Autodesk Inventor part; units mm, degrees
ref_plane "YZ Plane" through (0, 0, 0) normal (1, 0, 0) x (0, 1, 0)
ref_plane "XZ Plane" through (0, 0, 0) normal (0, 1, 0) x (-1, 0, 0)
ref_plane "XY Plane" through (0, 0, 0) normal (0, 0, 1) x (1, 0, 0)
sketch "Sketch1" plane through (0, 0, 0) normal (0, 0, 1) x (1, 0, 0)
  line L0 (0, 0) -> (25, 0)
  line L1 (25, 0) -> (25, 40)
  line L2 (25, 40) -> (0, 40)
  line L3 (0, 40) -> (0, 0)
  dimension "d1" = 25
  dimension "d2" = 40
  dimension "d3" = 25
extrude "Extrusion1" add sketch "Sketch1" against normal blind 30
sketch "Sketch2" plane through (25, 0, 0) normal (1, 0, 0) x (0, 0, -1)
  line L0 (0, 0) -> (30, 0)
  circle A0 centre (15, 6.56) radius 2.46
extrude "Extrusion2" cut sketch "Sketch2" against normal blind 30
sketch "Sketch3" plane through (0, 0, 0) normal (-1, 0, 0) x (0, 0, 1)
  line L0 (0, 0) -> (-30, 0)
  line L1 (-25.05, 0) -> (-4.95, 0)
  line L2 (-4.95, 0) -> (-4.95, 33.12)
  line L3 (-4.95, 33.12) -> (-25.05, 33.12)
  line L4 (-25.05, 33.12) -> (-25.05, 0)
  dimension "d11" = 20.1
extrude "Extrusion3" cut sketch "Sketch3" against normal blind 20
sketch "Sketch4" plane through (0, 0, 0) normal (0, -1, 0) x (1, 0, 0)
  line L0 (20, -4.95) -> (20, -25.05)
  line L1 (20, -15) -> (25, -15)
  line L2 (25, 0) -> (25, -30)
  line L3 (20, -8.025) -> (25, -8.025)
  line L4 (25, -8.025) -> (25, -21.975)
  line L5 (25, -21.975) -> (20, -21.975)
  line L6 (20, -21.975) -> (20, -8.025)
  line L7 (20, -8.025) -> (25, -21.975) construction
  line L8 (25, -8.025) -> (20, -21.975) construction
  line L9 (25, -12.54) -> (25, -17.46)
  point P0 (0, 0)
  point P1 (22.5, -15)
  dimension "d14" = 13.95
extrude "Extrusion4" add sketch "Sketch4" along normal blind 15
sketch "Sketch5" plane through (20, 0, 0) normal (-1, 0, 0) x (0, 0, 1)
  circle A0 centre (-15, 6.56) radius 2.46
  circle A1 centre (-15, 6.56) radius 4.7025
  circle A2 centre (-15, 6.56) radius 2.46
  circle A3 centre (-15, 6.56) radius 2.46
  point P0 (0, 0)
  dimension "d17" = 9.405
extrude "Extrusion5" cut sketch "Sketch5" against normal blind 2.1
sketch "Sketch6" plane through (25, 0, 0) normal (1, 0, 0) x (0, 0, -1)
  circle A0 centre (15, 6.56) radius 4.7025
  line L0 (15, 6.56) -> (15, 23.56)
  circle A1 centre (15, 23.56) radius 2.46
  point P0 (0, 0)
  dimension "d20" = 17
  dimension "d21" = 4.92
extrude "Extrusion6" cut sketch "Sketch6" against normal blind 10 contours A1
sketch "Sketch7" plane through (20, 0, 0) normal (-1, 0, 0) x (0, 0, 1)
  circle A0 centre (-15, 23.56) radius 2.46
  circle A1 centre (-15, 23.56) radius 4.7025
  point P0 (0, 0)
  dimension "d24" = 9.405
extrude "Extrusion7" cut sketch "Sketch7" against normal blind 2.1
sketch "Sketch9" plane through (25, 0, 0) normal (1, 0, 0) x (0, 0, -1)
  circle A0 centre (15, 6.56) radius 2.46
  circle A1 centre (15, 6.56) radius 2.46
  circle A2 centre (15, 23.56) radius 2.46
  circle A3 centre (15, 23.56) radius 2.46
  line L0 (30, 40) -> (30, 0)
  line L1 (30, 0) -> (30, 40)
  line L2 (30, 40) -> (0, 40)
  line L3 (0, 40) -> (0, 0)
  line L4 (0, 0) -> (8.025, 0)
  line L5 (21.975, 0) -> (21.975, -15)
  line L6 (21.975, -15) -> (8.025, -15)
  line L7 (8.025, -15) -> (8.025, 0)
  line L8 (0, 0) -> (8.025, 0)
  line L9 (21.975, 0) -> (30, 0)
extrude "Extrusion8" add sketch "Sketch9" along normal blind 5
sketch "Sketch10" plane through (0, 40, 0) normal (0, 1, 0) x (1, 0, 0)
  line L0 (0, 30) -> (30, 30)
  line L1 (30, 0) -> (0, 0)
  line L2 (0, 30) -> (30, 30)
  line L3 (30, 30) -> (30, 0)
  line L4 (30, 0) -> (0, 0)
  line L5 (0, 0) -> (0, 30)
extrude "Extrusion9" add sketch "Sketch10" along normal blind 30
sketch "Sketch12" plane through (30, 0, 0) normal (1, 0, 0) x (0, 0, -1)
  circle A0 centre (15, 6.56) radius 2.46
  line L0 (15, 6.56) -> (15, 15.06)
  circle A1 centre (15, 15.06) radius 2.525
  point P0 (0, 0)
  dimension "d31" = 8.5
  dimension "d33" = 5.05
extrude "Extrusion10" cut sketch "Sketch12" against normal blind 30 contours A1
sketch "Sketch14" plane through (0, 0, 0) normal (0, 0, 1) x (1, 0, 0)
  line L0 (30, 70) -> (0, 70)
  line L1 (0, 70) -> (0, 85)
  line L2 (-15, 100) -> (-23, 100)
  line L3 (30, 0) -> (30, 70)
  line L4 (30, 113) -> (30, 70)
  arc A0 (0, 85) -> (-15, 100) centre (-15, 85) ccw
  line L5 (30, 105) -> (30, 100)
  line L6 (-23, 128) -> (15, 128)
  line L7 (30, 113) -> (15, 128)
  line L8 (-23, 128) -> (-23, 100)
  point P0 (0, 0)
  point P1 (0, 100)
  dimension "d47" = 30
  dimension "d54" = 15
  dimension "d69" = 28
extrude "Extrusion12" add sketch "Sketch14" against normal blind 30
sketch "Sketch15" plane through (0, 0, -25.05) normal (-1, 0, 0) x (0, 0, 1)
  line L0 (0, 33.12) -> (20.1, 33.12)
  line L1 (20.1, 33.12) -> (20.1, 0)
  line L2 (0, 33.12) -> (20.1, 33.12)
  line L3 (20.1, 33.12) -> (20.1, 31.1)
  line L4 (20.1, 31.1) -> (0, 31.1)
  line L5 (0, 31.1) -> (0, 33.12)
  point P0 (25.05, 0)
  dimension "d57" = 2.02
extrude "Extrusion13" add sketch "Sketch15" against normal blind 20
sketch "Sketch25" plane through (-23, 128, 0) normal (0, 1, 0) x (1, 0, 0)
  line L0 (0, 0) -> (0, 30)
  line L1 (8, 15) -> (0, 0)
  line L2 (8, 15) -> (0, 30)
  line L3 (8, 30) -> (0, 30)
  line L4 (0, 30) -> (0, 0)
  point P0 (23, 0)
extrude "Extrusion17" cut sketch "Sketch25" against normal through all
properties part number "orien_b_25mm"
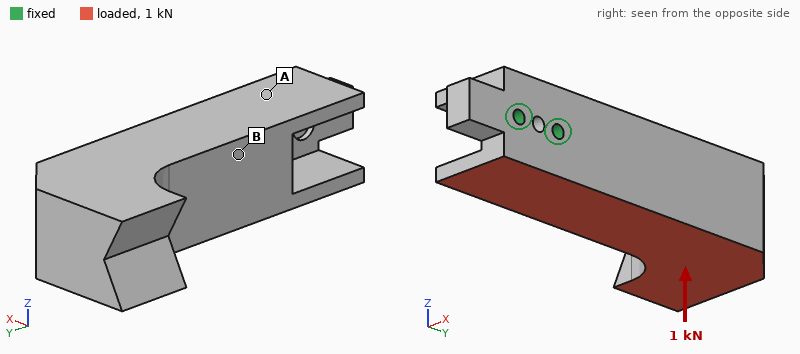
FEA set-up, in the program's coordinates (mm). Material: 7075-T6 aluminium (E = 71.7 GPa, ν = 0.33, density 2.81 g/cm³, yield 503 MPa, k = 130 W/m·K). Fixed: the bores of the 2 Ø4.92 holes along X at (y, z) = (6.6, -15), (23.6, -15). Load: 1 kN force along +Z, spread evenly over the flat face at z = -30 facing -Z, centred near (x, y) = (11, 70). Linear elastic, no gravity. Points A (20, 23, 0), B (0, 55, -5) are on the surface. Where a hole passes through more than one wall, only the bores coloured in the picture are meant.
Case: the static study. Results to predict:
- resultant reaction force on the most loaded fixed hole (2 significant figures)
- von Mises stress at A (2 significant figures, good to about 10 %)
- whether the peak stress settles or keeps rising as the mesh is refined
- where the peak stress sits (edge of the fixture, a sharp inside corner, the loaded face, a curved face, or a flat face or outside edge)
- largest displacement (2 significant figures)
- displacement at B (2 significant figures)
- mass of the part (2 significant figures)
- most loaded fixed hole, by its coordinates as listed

3.0 kN
19 MPa
keeps rising
edge of the fixture
0.12 mm
0.037 mm
330 g
(23.6, -15)
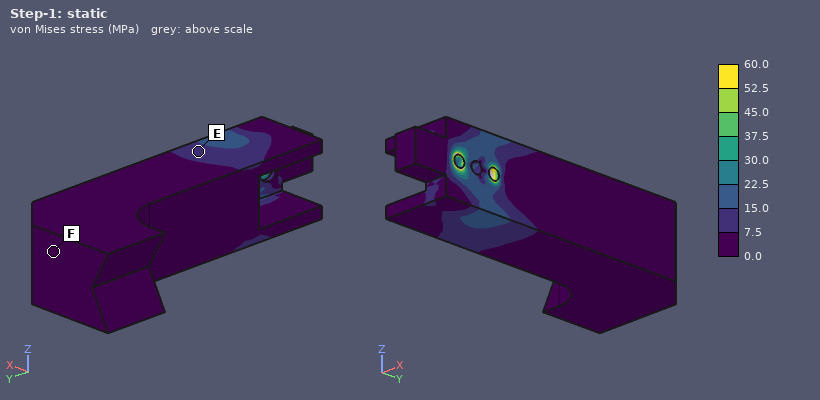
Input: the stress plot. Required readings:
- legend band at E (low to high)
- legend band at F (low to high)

7.5 to 15.0 MPa
0.0 to 7.5 MPa
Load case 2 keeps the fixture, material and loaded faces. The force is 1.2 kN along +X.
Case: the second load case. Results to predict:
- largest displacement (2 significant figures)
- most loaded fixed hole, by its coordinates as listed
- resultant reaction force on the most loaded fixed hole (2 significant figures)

0.19 mm
(23.6, -15)
3.3 kN
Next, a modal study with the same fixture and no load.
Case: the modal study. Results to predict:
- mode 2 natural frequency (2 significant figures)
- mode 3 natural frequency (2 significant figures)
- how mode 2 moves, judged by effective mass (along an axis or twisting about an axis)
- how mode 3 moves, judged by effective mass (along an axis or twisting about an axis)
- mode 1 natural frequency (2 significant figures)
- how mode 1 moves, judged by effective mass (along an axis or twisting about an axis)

990 Hz
2700 Hz
along Z
twisting about Y
840 Hz
along X
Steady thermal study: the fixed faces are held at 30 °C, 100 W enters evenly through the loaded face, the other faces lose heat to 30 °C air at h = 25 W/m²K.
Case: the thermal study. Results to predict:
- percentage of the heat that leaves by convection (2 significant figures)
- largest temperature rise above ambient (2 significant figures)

14 %
56 K
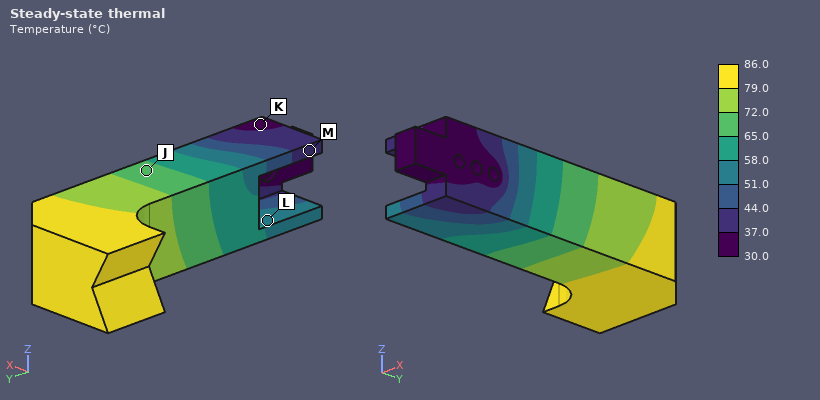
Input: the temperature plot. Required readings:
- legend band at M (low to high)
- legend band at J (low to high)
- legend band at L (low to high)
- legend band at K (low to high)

37.0 to 44.0 °C
65.0 to 72.0 °C
51.0 to 58.0 °C
30.0 to 37.0 °C
